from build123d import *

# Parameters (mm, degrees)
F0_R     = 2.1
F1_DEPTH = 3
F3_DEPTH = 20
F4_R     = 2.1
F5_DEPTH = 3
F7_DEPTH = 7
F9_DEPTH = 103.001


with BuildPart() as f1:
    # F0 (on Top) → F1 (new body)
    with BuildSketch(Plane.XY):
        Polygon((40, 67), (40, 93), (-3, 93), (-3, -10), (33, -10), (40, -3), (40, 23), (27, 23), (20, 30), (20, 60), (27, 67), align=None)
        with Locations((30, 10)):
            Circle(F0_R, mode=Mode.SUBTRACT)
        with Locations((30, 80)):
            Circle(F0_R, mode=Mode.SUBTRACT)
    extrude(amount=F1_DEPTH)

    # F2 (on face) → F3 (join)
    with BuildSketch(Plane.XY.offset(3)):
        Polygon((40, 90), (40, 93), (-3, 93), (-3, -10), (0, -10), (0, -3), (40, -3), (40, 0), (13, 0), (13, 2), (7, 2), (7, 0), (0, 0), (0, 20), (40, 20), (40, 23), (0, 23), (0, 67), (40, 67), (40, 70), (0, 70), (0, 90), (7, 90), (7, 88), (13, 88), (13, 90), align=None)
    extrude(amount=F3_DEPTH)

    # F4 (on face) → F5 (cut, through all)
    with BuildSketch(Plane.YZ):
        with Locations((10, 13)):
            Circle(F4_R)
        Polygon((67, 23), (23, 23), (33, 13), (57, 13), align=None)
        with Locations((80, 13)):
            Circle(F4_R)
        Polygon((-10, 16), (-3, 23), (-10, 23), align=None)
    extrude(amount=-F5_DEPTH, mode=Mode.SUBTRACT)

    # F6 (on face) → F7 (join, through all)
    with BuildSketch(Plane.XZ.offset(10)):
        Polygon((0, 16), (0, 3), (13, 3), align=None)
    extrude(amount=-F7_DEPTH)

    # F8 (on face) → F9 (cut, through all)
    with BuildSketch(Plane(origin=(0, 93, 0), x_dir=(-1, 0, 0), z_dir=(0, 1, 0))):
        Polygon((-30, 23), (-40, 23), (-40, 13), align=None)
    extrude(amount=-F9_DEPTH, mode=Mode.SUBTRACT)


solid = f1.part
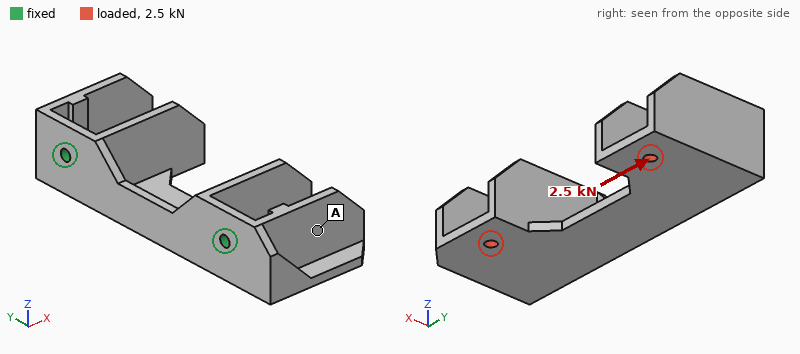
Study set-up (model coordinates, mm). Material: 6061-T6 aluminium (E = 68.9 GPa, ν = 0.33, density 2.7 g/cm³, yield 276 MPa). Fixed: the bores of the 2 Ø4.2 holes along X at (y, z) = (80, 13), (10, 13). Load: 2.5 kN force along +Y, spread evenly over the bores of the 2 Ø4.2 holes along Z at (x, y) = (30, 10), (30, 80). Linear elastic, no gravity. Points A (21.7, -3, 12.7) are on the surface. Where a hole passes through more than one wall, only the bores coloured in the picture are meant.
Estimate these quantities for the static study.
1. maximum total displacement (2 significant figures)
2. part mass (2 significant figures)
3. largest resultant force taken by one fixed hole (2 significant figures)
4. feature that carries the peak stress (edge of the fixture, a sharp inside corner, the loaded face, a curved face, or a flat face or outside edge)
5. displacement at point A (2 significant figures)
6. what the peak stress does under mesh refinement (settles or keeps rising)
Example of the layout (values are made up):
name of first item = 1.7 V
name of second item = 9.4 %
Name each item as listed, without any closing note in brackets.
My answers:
maximum total displacement = 0.35 mm
part mass = 69 g
largest resultant force taken by one fixed hole = 1.7 kN
feature that carries the peak stress = edge of the fixture
displacement at point A = 0.19 mm
what the peak stress does under mesh refinement = keeps rising
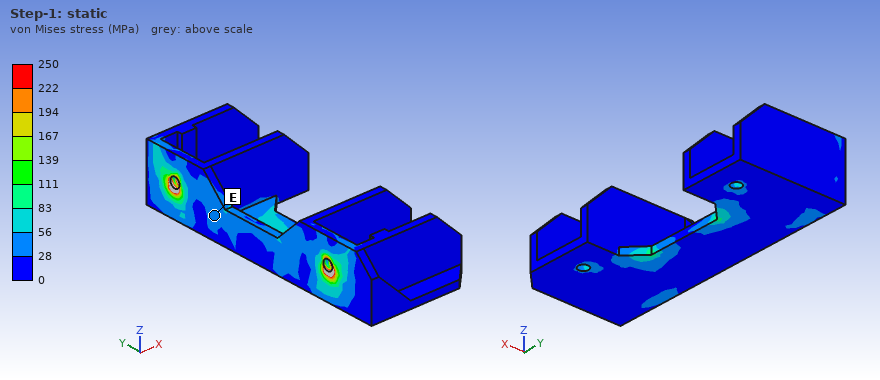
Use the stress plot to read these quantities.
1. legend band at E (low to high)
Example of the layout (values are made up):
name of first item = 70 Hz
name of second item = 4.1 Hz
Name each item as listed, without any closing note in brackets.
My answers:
legend band at E = 28 to 56 MPa
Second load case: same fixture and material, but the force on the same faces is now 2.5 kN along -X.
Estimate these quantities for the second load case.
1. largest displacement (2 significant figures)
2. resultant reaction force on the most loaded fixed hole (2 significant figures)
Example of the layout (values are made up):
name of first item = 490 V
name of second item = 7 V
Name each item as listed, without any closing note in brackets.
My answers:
largest displacement = 0.44 mm
resultant reaction force on the most loaded fixed hole = 1.3 kN
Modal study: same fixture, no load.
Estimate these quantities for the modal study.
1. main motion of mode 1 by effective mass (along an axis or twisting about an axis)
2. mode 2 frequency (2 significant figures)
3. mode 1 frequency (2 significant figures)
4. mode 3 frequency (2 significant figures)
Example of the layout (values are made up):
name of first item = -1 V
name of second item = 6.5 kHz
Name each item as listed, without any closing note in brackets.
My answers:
main motion of mode 1 by effective mass = along Z
mode 2 frequency = 1700 Hz
mode 1 frequency = 1500 Hz
mode 3 frequency = 3300 Hz
